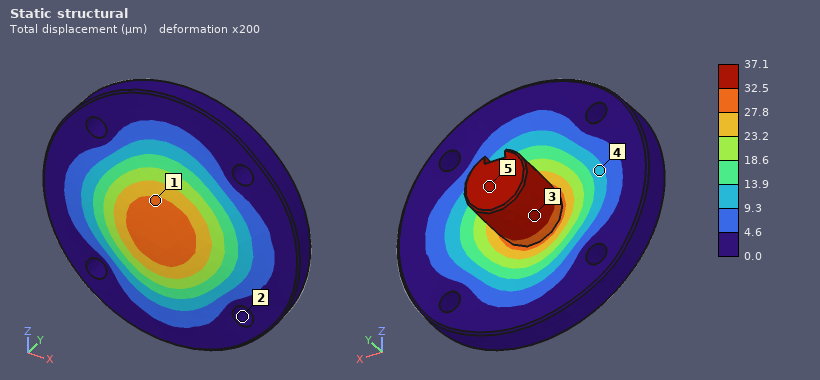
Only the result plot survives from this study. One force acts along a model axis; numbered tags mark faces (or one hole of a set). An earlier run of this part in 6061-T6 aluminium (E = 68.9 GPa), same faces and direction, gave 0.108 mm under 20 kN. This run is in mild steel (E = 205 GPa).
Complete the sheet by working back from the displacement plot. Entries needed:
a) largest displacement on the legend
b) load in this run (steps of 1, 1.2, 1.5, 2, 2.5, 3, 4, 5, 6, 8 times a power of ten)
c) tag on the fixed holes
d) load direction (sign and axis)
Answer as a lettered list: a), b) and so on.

a) 37.1 µm
b) 20 kN
c) 2
d) -Y
